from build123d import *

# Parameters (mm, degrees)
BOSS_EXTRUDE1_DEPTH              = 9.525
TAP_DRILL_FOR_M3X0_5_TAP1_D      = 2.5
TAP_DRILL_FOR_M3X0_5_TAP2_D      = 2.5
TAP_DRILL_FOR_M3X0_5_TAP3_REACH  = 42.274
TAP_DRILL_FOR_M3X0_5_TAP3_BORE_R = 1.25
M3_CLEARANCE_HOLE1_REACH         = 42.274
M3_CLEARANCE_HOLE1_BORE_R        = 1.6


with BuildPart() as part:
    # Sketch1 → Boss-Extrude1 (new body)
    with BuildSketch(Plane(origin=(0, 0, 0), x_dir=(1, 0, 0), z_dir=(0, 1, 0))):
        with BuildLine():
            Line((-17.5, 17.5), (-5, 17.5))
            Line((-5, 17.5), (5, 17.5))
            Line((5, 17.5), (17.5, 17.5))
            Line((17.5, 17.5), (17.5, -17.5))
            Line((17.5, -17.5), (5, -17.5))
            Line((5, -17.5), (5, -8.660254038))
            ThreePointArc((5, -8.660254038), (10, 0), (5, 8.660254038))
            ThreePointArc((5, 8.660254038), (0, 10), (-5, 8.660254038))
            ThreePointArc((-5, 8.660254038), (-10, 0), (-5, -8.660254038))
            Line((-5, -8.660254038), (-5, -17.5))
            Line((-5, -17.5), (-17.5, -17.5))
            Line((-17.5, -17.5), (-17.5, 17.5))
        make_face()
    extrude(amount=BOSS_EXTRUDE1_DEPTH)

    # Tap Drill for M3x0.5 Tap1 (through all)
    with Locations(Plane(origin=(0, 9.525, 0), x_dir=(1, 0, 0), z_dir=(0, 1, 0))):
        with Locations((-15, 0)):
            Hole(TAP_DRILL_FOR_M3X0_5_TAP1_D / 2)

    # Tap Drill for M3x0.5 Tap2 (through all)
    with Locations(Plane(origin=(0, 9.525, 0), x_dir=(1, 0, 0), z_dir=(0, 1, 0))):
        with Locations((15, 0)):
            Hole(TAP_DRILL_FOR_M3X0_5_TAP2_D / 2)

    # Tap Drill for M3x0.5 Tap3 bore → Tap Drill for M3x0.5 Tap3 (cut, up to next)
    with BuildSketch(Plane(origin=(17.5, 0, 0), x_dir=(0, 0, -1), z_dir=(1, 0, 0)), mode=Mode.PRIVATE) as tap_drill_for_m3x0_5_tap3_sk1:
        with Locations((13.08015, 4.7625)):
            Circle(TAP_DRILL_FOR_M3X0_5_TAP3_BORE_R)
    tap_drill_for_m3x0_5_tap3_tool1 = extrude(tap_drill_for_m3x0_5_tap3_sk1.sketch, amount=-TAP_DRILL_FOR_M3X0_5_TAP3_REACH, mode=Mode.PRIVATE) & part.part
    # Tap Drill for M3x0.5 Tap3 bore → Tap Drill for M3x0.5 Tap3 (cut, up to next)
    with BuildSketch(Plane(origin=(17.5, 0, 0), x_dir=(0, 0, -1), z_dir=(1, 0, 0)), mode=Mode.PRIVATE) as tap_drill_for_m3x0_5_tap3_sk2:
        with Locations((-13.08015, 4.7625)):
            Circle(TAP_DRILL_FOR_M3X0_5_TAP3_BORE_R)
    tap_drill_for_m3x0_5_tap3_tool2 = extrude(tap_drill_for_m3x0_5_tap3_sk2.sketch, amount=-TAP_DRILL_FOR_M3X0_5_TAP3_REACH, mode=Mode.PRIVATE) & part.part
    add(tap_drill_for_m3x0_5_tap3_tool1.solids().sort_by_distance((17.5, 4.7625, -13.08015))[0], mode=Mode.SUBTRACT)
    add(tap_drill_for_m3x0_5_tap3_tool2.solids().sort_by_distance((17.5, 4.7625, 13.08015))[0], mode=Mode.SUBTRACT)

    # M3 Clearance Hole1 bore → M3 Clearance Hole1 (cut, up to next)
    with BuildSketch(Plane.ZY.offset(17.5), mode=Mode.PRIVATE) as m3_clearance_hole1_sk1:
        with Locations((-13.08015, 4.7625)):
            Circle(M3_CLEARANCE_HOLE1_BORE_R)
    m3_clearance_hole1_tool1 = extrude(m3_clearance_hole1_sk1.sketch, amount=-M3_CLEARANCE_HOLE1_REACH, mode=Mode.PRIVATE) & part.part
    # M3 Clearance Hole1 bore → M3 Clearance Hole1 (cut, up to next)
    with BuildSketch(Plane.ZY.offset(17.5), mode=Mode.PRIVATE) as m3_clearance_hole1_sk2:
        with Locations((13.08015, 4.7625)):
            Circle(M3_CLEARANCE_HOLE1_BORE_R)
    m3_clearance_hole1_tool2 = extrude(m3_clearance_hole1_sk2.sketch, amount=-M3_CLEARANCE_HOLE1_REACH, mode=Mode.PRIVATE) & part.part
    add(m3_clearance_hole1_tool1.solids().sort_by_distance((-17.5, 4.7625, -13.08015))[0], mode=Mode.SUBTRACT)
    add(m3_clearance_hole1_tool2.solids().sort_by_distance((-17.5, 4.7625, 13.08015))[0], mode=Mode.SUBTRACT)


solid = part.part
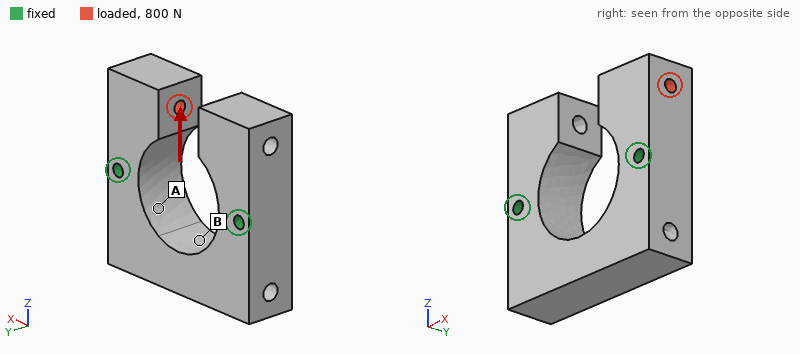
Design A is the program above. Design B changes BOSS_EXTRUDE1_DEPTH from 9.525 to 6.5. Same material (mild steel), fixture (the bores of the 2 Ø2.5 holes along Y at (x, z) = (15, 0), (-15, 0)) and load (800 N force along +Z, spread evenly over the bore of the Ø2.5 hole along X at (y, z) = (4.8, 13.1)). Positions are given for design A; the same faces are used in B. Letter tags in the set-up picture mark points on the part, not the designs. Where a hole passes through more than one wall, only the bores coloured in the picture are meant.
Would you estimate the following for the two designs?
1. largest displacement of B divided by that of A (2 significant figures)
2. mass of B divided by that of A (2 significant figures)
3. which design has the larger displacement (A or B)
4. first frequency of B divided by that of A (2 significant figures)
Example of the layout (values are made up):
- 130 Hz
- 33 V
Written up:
- 1.9
- 0.66
- B
- 0.90
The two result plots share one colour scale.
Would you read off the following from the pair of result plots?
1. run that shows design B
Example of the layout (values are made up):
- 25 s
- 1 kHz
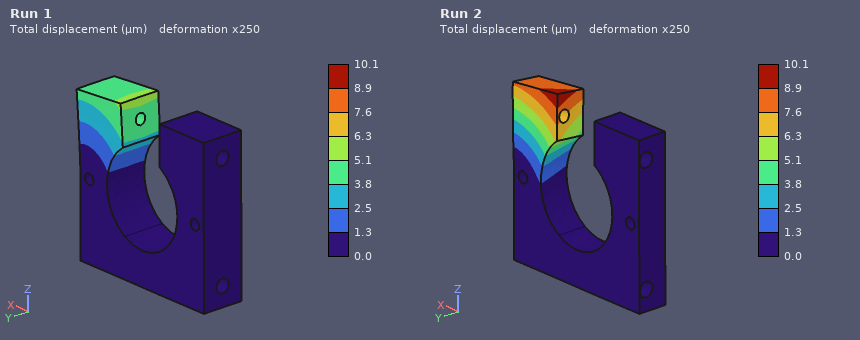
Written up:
- Run 2
